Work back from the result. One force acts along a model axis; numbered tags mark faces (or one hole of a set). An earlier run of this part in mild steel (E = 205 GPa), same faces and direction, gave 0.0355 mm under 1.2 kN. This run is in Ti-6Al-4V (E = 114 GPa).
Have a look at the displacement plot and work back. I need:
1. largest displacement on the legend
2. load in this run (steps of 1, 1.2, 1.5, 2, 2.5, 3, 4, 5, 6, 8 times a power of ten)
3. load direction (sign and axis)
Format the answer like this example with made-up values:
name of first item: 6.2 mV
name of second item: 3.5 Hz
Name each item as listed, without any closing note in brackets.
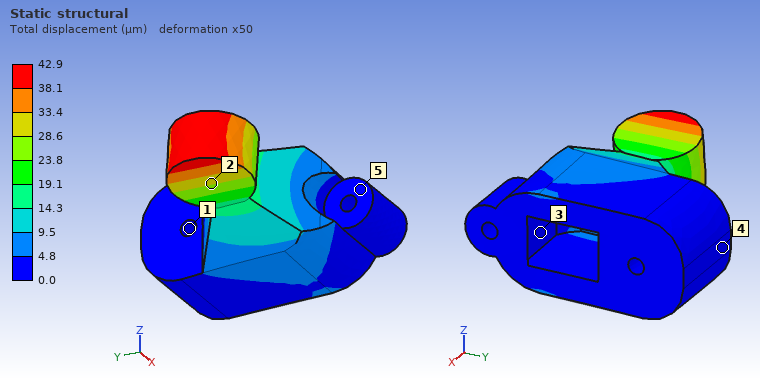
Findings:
largest displacement on the legend: 42.9 µm
load in this run: 800 N
load direction: +Z
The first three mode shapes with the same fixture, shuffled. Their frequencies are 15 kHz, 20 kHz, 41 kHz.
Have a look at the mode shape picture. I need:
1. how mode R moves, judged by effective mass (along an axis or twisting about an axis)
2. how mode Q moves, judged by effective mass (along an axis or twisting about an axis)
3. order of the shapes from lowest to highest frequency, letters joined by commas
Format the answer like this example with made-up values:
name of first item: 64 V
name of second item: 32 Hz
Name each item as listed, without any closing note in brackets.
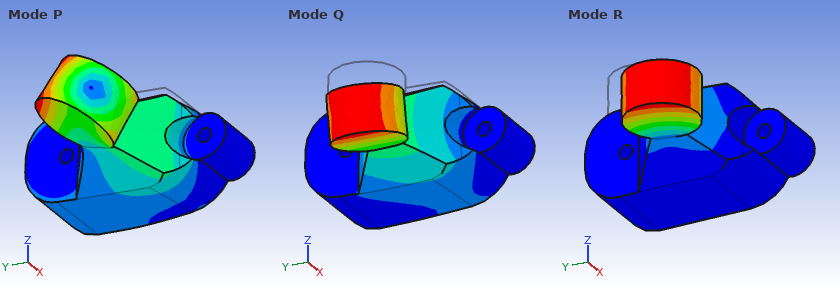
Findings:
how mode R moves, judged by effective mass: along Y
how mode Q moves, judged by effective mass: along Z
order of the shapes from lowest to highest frequency, letters joined by commas: Q, R, P
